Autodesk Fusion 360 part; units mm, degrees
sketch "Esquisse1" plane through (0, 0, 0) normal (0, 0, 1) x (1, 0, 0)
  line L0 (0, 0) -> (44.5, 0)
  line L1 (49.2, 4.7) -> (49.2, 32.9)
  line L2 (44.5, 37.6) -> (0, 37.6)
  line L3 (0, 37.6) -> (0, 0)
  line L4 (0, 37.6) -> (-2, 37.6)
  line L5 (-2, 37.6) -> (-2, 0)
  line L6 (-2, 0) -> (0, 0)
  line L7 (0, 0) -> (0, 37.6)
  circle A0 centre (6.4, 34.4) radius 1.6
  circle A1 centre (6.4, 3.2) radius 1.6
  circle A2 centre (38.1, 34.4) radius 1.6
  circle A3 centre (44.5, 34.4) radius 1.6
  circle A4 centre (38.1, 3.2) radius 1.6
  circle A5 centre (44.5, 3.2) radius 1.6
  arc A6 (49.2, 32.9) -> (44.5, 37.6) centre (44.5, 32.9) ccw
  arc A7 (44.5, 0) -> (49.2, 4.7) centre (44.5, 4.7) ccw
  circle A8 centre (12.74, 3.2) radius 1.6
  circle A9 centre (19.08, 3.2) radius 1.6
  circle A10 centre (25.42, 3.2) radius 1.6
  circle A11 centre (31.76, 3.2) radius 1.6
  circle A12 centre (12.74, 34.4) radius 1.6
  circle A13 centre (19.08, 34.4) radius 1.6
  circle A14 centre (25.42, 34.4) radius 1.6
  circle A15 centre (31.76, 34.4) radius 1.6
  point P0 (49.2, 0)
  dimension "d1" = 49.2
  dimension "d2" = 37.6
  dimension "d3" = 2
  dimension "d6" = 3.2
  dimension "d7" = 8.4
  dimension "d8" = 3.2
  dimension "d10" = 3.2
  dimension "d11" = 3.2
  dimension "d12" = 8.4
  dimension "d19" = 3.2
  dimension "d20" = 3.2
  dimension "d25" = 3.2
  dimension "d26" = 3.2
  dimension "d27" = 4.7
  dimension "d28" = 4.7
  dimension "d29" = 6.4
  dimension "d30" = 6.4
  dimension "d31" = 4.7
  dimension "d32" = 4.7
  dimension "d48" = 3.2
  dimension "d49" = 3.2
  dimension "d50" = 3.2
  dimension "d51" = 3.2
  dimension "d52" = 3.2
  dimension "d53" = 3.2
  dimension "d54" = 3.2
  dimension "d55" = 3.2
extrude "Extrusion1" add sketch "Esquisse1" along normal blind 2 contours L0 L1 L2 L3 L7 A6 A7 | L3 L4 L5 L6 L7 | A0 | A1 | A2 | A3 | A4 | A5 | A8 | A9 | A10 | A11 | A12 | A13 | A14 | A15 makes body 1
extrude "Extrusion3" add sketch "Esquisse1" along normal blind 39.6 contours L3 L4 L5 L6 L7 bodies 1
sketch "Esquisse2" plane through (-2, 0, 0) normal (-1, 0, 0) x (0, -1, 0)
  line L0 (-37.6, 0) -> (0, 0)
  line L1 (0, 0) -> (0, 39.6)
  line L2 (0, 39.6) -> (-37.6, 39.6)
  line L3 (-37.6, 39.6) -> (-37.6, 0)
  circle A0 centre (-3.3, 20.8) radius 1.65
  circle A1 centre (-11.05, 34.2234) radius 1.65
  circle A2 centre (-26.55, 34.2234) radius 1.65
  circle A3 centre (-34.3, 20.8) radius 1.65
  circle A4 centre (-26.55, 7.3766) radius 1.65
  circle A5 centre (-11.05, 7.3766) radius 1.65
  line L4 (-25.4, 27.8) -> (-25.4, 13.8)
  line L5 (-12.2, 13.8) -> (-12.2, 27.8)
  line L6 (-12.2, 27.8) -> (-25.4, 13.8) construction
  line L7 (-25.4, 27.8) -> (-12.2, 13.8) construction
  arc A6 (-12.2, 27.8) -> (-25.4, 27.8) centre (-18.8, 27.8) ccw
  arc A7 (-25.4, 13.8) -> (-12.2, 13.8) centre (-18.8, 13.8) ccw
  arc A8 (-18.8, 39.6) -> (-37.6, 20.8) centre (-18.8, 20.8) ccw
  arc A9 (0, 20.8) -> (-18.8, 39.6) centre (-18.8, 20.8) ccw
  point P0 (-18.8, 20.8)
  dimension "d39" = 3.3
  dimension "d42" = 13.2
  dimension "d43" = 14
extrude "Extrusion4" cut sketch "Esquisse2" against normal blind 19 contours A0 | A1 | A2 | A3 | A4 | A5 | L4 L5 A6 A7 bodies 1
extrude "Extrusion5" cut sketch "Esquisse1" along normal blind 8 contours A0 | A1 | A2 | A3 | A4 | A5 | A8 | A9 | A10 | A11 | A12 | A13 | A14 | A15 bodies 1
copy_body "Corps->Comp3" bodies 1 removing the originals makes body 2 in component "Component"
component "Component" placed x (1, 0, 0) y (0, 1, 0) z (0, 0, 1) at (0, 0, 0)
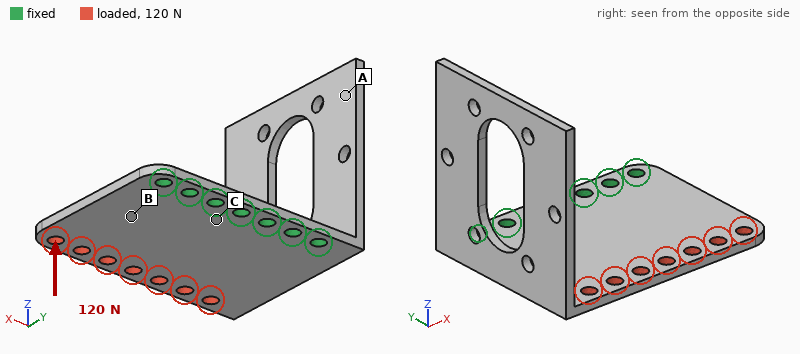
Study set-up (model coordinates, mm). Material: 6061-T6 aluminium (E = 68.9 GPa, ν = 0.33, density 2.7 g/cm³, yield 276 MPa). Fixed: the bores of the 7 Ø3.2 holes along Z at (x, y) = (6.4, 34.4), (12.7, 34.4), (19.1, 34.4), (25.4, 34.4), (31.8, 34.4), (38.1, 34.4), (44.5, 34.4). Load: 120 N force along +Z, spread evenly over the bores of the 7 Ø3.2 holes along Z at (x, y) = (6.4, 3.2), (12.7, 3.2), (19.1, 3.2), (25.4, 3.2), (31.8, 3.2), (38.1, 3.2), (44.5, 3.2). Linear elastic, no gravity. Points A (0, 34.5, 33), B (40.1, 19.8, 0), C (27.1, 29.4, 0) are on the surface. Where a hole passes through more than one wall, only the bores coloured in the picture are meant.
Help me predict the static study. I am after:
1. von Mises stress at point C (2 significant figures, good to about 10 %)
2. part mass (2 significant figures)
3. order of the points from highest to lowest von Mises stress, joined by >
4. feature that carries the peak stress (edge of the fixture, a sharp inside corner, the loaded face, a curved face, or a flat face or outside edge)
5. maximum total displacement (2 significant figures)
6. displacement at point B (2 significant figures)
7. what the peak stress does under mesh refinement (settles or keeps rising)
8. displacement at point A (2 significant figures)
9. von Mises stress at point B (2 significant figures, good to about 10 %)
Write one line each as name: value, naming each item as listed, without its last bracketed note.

von Mises stress at point C: 71 MPa
part mass: 15 g
order of the points from highest to lowest von Mises stress, joined by >: C > B > A
feature that carries the peak stress: edge of the fixture
maximum total displacement: 0.44 mm
displacement at point B: 0.100 mm
what the peak stress does under mesh refinement: keeps rising
displacement at point A: 0.23 mm
von Mises stress at point B: 45 MPa
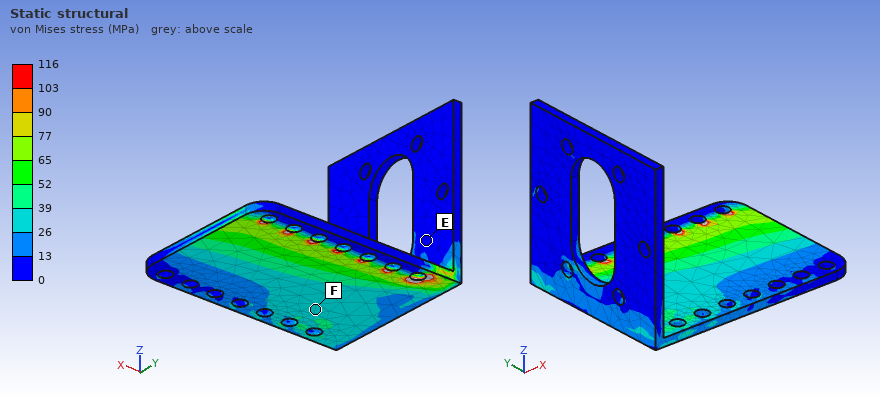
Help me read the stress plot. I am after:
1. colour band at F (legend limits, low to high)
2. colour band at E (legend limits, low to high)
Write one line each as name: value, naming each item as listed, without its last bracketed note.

colour band at F: 26 to 39 MPa
colour band at E: 0 to 13 MPa
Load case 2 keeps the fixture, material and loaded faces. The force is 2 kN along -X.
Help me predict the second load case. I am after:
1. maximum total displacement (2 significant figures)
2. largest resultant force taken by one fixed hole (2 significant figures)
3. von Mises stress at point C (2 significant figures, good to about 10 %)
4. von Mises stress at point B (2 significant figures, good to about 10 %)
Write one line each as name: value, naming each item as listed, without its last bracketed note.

maximum total displacement: 56 µm
largest resultant force taken by one fixed hole: 1.3 kN
von Mises stress at point C: 48 MPa
von Mises stress at point B: 41 MPa
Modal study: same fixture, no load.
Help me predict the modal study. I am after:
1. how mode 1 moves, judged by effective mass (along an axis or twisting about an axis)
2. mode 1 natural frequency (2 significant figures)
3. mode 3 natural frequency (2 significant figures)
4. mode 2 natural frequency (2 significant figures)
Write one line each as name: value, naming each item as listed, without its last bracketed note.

how mode 1 moves, judged by effective mass: along X
mode 1 natural frequency: 740 Hz
mode 3 natural frequency: 2000 Hz
mode 2 natural frequency: 1000 Hz
